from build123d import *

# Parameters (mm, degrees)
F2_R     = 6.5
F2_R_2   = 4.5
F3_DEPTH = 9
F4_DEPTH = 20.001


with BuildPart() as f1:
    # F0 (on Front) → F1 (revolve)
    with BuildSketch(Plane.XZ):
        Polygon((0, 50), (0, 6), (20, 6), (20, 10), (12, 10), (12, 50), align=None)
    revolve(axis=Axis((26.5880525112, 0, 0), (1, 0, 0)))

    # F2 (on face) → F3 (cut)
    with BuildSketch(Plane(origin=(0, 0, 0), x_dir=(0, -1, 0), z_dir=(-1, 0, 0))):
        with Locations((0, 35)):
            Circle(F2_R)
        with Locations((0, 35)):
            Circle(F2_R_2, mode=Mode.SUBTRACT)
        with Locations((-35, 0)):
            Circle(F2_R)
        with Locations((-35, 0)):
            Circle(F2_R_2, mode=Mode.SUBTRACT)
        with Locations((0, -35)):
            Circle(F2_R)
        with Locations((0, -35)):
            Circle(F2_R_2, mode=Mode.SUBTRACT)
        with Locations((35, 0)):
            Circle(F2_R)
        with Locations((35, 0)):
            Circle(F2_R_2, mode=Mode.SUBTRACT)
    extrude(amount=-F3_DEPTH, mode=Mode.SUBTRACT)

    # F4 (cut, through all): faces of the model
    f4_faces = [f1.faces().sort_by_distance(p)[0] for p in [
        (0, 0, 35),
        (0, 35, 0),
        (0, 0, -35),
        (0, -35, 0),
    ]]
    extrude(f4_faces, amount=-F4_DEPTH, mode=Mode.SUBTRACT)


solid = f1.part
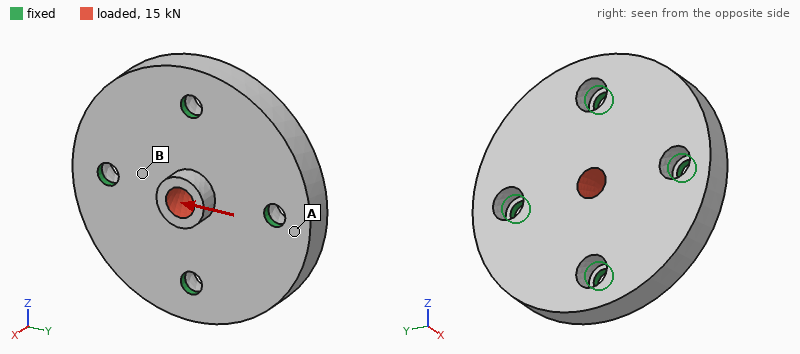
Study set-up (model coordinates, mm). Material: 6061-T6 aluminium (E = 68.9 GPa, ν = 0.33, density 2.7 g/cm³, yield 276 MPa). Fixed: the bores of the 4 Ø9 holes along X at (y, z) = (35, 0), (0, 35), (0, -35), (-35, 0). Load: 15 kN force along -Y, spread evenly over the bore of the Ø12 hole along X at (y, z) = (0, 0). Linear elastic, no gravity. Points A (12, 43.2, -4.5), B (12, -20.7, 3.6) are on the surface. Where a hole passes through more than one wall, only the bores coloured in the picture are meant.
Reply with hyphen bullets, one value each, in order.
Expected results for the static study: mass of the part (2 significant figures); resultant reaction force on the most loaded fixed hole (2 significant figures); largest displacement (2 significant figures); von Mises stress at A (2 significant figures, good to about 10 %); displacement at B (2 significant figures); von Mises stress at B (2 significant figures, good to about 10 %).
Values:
- 240 g
- 4.2 kN
- 34 µm
- 17 MPa
- 8.5 µm
- 37 MPa
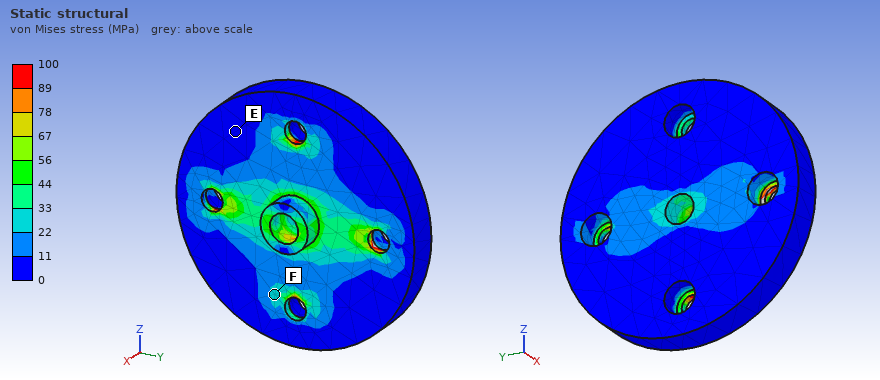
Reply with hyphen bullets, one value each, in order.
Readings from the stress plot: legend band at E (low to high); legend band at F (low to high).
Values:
- 0 to 11 MPa
- 22 to 33 MPa
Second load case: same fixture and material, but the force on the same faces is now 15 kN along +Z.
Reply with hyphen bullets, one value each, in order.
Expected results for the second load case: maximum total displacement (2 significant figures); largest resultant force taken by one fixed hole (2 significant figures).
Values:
- 34 µm
- 4.2 kN
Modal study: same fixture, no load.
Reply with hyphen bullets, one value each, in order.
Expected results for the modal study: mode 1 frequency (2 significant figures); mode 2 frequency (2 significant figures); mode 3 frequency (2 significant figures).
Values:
- 8400 Hz
- 9300 Hz
- 9300 Hz
